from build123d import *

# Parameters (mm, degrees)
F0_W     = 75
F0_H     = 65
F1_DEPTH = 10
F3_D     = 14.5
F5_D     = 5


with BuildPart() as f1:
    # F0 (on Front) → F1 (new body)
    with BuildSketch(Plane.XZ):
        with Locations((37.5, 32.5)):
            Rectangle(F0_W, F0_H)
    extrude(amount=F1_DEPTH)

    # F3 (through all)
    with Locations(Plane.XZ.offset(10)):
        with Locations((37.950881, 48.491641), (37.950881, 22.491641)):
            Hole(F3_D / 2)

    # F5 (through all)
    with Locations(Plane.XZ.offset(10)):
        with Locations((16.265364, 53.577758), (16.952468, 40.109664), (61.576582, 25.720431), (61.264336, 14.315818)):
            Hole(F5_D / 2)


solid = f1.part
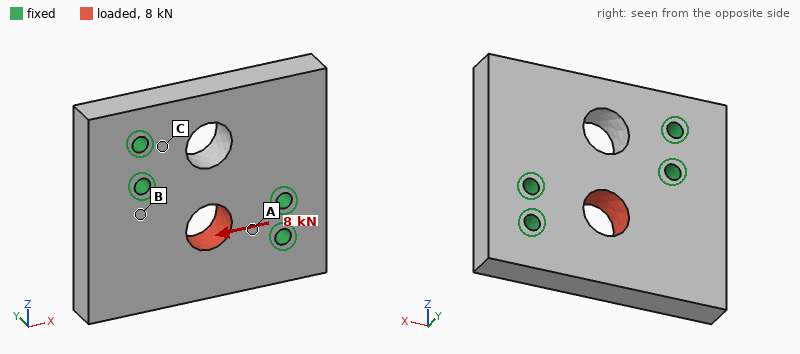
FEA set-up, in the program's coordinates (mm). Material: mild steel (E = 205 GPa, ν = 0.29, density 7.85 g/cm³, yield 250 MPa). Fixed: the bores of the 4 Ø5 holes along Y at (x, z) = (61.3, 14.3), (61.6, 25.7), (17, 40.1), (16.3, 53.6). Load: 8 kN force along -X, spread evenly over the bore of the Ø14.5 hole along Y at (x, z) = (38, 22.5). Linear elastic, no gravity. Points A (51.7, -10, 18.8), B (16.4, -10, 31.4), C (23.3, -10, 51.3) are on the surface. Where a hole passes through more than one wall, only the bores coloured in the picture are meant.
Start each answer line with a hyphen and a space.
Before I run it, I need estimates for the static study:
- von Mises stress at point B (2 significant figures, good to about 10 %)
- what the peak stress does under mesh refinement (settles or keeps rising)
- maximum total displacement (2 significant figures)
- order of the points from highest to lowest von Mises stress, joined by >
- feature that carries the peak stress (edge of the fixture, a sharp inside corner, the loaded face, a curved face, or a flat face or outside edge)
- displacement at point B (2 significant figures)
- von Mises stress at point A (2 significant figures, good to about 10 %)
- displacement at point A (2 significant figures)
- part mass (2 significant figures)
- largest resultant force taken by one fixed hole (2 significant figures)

- 11 MPa
- keeps rising
- 3.0 µm
- A > B > C
- edge of the fixture
- 1.1 µm
- 22 MPa
- 0.83 µm
- 350 g
- 3.0 kN
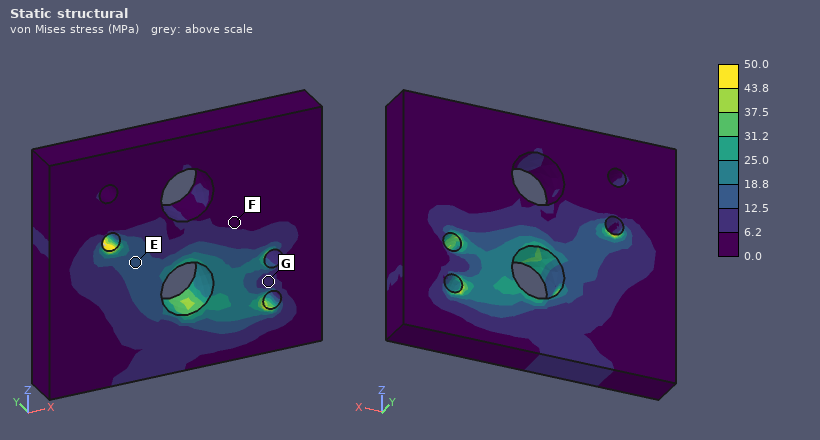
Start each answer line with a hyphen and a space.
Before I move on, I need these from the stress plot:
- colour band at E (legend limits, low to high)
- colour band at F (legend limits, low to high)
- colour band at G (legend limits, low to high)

- 12.5 to 18.8 MPa
- 0.0 to 6.2 MPa
- 6.2 to 12.5 MPa
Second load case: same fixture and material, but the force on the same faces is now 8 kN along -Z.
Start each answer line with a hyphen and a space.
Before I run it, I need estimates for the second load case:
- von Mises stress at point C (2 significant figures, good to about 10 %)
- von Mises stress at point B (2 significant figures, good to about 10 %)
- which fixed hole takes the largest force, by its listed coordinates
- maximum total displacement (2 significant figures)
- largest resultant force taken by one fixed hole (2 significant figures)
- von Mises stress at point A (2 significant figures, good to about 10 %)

- 13 MPa
- 16 MPa
- (17, 40.1)
- 3.6 µm
- 2.9 kN
- 21 MPa
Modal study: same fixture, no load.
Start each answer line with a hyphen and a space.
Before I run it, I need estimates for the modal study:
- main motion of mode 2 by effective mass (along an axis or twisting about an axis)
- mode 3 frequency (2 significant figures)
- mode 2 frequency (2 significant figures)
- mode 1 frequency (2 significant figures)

- along Y
- 14 kHz
- 6500 Hz
- 5800 Hz
